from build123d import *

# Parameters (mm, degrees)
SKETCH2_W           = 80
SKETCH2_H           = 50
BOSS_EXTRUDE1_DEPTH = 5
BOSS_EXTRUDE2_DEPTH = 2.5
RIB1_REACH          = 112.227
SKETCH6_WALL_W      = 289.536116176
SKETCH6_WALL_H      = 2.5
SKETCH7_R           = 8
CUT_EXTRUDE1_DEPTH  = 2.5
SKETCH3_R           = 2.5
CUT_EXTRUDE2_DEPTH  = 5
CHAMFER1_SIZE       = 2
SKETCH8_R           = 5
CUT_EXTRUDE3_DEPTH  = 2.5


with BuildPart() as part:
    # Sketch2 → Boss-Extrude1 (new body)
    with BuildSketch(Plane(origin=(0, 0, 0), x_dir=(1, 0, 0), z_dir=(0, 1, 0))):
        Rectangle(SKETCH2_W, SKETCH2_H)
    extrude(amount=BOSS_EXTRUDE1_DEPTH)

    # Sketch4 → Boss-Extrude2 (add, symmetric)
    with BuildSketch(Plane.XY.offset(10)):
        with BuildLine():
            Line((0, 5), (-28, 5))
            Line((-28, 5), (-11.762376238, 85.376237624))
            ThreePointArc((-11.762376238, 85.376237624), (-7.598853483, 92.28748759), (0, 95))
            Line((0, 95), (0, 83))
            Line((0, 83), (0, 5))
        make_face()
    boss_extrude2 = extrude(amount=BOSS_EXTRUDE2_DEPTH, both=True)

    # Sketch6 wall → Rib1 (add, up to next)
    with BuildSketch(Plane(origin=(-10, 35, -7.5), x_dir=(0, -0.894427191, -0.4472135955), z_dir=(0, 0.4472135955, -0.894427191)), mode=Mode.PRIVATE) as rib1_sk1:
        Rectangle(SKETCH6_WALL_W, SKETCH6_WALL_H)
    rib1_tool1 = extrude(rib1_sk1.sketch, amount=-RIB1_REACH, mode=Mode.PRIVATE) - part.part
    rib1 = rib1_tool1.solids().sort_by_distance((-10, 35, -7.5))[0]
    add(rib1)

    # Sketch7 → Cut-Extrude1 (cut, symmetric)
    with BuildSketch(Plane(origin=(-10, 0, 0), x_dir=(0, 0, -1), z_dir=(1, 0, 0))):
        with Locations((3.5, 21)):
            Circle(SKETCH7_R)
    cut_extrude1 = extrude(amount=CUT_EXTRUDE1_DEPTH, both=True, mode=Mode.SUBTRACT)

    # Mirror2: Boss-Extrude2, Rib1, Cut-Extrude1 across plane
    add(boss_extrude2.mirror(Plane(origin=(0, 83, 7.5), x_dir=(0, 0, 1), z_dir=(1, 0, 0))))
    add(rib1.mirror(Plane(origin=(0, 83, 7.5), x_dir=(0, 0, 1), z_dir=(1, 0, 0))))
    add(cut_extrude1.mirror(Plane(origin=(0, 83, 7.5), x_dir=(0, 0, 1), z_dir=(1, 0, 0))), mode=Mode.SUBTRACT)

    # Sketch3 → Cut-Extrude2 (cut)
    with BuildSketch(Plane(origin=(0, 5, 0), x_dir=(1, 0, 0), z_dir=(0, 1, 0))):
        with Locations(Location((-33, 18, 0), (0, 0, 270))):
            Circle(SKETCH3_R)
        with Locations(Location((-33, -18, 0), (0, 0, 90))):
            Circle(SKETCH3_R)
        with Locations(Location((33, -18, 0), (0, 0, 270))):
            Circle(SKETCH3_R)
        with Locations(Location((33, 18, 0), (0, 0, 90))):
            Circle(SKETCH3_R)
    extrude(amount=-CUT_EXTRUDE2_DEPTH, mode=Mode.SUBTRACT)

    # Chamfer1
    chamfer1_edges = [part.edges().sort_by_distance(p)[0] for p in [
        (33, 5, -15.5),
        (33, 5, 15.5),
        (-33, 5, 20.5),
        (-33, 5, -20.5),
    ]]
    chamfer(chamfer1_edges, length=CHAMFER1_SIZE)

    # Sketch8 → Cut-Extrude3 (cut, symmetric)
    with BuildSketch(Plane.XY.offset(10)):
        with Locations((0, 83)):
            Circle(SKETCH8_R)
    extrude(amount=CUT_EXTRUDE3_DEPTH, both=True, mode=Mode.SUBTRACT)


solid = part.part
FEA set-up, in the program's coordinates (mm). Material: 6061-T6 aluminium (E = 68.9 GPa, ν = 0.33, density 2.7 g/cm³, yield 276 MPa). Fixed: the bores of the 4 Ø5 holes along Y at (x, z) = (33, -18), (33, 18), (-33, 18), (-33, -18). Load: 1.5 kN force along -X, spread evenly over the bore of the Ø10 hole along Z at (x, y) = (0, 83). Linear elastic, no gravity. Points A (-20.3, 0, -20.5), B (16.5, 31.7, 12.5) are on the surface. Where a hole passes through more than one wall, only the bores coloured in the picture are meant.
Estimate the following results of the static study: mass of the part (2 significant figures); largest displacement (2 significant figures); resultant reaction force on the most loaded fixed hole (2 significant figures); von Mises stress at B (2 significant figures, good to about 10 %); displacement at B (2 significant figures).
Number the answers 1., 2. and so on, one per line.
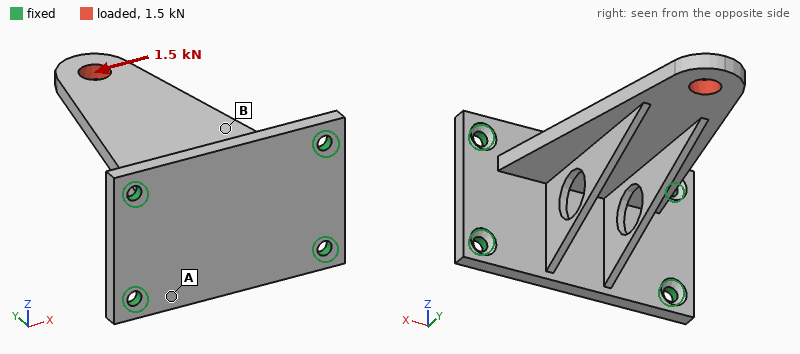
1. 110 g
2. 0.24 mm
3. 1.9 kN
4. 34 MPa
5. 0.056 mm
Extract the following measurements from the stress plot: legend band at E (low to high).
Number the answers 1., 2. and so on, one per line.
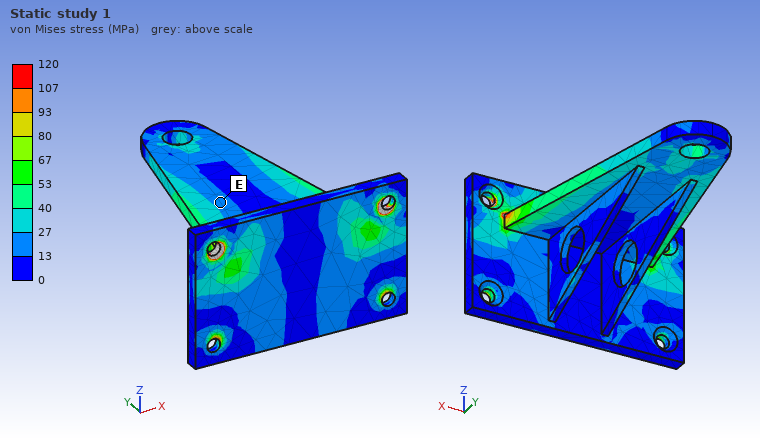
1. 13 to 27 MPa
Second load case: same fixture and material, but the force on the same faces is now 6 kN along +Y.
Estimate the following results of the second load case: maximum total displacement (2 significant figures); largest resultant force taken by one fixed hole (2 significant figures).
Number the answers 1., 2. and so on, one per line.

1. 0.19 mm
2. 2.9 kN
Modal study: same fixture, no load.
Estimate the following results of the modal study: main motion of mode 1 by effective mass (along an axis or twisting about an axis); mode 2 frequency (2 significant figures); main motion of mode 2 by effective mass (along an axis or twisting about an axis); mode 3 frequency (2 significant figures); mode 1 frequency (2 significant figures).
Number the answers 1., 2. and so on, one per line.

1. along Z
2. 3700 Hz
3. along X
4. 4200 Hz
5. 1500 Hz
